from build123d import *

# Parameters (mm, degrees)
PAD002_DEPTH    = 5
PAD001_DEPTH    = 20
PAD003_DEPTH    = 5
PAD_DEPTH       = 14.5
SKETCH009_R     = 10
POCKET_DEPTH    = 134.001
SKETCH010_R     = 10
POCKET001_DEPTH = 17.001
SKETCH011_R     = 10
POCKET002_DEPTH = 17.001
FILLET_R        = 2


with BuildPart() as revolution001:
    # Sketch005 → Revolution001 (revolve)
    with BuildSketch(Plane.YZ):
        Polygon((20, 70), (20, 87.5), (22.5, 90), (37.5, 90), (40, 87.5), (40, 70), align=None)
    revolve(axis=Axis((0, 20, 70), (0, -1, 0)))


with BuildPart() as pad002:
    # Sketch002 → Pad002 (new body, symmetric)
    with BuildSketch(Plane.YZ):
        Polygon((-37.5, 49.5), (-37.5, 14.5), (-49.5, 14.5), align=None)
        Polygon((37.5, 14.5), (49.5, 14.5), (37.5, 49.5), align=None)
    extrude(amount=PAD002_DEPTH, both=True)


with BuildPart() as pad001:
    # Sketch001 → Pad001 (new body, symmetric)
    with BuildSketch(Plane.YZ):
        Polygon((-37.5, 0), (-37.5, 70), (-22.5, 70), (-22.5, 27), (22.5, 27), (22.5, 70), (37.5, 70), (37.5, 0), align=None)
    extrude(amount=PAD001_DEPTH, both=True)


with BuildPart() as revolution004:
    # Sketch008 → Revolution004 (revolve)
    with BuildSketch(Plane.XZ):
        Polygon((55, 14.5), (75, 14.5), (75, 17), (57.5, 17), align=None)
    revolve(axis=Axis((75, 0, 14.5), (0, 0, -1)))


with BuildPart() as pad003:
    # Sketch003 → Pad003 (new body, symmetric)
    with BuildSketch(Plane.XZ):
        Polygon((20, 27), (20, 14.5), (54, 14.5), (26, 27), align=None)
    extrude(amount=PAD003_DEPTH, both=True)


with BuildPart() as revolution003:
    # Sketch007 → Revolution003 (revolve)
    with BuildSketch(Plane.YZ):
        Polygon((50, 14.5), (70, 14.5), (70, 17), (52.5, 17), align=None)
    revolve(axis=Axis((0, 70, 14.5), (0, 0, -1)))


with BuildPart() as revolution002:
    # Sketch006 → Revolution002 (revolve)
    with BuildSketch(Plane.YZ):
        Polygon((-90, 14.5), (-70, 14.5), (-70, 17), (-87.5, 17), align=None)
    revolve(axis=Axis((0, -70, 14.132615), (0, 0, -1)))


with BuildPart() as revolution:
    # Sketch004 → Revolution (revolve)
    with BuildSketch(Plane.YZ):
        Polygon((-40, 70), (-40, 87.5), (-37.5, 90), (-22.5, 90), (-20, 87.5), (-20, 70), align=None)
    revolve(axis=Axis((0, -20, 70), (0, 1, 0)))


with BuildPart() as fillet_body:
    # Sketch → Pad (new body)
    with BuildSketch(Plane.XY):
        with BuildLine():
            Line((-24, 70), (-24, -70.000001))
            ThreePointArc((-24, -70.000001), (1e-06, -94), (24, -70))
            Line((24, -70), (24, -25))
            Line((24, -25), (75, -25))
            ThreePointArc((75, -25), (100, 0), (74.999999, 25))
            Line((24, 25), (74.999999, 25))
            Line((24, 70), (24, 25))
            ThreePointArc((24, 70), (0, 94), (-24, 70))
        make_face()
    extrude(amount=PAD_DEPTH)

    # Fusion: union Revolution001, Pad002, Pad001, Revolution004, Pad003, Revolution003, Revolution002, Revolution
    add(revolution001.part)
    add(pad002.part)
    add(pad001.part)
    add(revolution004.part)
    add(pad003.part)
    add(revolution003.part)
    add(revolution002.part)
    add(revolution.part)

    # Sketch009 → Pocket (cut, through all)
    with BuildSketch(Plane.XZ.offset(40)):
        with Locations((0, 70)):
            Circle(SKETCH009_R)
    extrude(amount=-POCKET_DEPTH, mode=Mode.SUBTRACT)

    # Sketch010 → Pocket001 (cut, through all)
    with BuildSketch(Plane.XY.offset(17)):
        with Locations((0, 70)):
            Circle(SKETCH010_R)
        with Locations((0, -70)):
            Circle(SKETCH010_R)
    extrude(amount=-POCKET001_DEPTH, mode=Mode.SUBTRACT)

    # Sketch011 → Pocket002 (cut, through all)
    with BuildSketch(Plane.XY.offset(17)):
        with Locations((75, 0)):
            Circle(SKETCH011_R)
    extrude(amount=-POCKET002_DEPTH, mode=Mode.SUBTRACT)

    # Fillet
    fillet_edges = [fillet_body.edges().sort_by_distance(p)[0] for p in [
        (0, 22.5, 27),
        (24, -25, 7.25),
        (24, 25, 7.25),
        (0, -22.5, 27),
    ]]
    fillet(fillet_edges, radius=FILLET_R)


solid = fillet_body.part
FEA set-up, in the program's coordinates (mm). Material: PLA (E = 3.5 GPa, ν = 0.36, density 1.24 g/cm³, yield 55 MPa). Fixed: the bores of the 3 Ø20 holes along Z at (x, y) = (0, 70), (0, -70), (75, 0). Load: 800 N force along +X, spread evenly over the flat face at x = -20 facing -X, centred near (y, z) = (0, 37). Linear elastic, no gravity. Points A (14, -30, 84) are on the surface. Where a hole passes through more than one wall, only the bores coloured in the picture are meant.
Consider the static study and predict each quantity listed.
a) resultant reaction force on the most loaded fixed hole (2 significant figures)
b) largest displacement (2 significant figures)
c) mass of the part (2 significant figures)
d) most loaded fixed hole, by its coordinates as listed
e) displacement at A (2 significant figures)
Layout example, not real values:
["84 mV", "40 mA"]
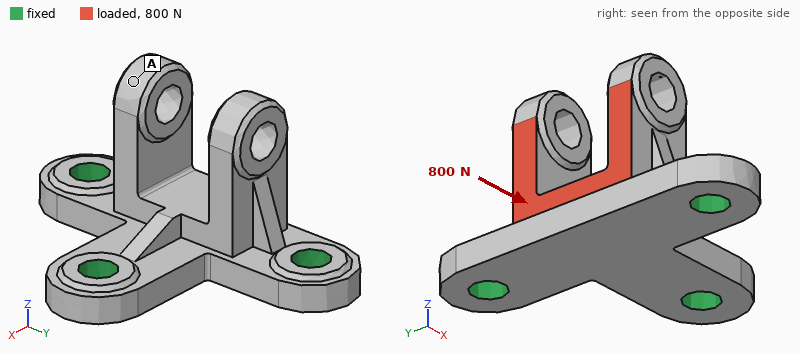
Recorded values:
["550 N", "0.21 mm", "350 g", "(75, 0)", "0.20 mm"]
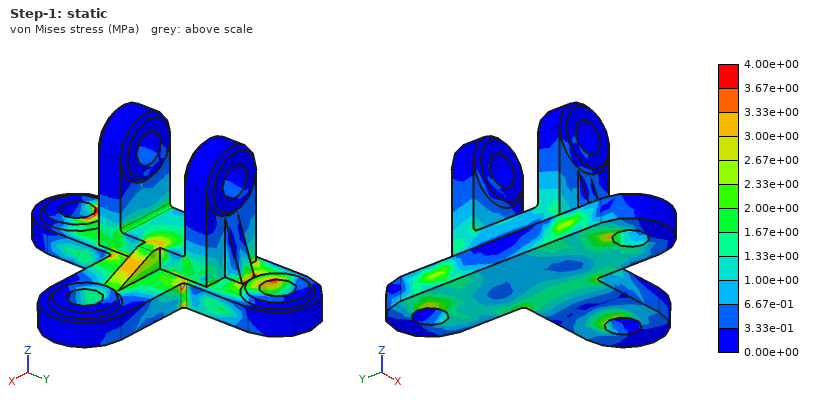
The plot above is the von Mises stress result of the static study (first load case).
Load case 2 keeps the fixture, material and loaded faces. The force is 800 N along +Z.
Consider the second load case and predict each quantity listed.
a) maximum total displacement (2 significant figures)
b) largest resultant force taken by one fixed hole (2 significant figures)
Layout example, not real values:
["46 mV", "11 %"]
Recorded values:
["0.22 mm", "500 N"]
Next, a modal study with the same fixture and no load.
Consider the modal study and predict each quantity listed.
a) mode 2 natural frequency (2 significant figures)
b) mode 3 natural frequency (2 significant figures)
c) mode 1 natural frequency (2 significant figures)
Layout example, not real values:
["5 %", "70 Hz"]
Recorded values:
["1000 Hz", "1000 Hz", "840 Hz"]
